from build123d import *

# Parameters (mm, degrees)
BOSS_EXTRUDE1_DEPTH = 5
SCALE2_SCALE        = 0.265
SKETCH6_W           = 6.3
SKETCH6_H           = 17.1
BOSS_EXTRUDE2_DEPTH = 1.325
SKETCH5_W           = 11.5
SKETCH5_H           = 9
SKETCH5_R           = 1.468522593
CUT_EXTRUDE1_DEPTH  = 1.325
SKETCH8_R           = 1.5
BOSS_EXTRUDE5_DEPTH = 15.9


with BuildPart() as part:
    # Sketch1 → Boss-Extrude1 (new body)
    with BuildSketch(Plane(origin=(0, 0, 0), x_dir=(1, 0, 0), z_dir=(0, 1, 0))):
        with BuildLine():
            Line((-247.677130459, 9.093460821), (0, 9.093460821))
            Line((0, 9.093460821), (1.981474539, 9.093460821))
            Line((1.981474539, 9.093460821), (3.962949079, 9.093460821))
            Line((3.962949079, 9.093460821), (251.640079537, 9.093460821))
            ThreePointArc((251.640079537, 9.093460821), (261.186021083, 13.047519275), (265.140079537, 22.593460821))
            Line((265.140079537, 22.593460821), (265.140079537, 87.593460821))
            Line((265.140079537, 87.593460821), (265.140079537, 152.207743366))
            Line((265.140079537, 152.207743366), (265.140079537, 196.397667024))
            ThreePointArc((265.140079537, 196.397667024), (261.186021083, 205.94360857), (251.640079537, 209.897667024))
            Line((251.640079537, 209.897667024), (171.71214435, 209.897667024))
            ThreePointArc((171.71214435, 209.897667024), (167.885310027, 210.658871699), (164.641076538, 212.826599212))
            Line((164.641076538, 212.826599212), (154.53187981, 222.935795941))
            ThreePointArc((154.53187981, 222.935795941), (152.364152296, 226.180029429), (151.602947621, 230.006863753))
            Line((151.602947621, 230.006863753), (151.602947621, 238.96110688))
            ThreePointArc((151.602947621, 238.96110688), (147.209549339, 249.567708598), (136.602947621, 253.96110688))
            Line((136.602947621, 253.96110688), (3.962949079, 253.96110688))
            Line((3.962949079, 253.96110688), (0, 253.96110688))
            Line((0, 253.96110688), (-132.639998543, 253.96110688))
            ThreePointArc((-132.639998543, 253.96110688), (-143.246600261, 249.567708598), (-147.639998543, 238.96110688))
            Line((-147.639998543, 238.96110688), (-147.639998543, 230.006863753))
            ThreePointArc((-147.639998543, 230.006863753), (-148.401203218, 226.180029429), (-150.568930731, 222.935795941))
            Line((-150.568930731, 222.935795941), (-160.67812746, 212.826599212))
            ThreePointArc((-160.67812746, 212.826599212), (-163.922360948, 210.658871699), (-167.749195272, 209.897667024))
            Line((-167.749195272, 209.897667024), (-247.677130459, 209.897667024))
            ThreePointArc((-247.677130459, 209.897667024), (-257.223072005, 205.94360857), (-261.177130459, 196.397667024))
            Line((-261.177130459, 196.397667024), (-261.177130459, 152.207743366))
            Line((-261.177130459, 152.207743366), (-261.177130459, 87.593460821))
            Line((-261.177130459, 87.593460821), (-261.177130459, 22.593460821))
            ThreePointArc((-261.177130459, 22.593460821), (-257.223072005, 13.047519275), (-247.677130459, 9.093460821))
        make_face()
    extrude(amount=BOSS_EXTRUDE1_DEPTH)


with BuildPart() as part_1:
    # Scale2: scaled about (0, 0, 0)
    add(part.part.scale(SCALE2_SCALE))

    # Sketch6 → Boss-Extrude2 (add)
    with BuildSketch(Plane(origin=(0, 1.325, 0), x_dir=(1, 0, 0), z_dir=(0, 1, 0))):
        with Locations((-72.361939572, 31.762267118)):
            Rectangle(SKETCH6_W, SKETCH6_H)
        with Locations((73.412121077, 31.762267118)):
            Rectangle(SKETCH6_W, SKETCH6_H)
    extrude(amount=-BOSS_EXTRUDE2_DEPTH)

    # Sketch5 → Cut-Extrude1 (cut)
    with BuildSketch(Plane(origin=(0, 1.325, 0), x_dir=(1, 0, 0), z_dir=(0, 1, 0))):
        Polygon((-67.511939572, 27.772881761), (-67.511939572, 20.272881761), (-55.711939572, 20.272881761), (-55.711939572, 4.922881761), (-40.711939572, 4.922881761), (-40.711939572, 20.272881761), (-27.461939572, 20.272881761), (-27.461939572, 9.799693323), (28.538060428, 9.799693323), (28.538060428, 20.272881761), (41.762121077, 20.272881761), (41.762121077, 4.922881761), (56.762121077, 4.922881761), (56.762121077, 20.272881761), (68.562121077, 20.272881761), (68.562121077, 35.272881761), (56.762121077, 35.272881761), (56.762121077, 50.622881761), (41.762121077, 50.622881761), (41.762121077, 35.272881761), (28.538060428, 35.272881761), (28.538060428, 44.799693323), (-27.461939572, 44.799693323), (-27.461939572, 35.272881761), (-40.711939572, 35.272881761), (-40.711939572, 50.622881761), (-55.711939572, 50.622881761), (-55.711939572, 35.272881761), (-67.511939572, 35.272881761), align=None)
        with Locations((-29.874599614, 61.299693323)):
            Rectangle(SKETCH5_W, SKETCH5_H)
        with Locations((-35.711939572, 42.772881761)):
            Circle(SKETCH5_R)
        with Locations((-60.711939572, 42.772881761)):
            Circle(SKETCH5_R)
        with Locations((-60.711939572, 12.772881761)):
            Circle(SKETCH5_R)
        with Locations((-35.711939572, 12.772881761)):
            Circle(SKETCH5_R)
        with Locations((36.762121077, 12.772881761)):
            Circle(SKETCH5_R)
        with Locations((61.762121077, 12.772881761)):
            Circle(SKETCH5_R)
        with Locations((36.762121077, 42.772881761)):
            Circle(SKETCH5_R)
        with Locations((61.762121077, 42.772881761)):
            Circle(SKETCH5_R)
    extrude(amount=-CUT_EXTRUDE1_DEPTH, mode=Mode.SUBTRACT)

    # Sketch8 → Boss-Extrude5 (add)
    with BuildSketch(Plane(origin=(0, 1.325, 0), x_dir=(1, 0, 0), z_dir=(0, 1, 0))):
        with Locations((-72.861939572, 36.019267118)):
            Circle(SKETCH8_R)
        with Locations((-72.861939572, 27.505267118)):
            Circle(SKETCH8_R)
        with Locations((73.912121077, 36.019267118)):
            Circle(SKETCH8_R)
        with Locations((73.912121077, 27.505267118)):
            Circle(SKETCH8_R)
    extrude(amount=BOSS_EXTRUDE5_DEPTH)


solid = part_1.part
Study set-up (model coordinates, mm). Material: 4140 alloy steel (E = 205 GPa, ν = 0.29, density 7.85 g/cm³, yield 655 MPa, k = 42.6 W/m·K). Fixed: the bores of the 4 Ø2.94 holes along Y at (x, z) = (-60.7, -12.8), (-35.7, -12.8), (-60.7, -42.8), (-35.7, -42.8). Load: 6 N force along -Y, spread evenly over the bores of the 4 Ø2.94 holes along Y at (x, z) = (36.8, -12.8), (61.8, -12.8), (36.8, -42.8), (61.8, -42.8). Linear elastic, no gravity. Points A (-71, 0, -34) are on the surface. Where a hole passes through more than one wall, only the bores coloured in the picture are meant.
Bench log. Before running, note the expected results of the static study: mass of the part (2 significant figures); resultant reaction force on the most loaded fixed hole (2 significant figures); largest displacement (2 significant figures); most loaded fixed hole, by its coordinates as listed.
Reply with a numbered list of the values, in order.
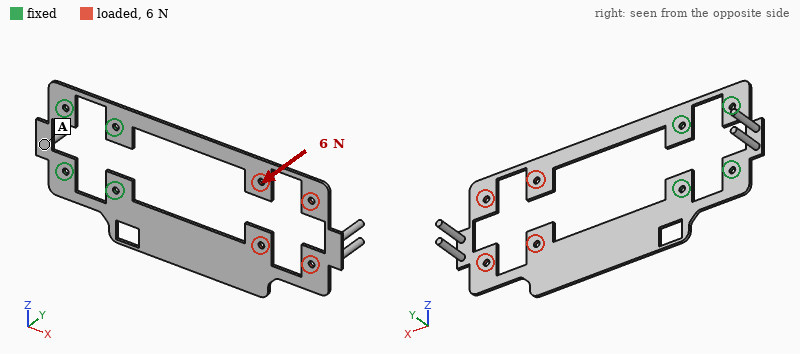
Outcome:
1. 49 g
2. 7.0 N
3. 1.9 mm
4. (-35.7, -42.8)
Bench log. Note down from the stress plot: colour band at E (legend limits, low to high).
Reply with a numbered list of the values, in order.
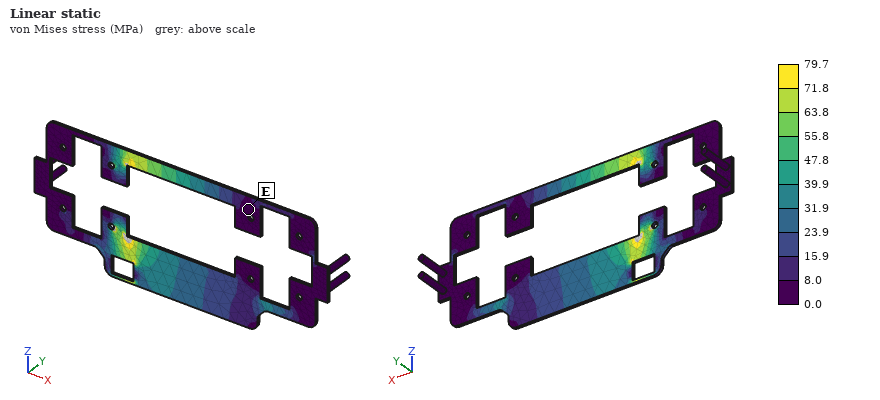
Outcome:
1. 0.0 to 8.0 MPa
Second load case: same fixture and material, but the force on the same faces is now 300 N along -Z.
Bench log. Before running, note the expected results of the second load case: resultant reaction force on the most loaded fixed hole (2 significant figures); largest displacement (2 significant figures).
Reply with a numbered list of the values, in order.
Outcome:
1. 910 N
2. 1.1 mm
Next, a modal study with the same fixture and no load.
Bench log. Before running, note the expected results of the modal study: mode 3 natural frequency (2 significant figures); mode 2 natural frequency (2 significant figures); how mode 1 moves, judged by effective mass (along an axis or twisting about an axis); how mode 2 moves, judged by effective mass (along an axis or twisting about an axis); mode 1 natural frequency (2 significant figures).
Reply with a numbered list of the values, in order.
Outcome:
1. 390 Hz
2. 220 Hz
3. along Y
4. twisting about X
5. 76 Hz
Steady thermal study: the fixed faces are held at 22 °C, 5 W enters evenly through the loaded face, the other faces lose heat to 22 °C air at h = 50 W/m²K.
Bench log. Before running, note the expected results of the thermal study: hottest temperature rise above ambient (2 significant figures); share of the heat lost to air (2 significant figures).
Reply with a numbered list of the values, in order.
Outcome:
1. 40 K
2. 98 %
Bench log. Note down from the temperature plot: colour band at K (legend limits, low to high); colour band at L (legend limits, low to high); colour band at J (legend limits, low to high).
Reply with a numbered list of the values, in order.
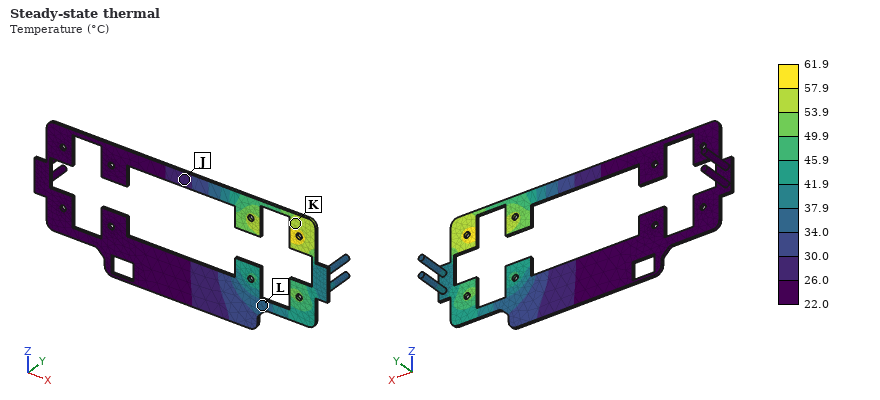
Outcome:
1. 53.9 to 57.9 °C
2. 34.0 to 37.9 °C
3. 26.0 to 30.0 °C
